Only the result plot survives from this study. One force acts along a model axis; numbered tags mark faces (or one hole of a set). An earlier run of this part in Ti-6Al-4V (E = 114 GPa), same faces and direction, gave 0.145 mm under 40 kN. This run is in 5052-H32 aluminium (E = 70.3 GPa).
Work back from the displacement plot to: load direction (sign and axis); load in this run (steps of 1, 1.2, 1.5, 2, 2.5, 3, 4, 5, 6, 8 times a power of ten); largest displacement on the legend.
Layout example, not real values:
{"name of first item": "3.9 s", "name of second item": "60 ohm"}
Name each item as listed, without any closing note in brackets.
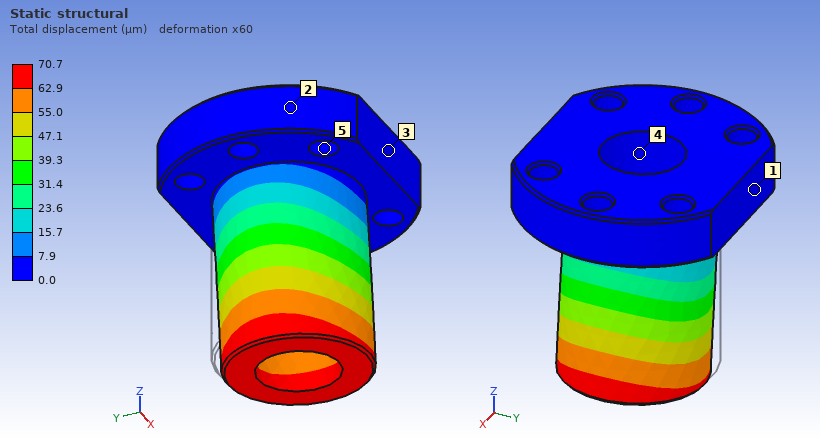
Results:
{"load direction": "+X", "load in this run": "12 kN", "largest displacement on the legend": "70.7 µm"}
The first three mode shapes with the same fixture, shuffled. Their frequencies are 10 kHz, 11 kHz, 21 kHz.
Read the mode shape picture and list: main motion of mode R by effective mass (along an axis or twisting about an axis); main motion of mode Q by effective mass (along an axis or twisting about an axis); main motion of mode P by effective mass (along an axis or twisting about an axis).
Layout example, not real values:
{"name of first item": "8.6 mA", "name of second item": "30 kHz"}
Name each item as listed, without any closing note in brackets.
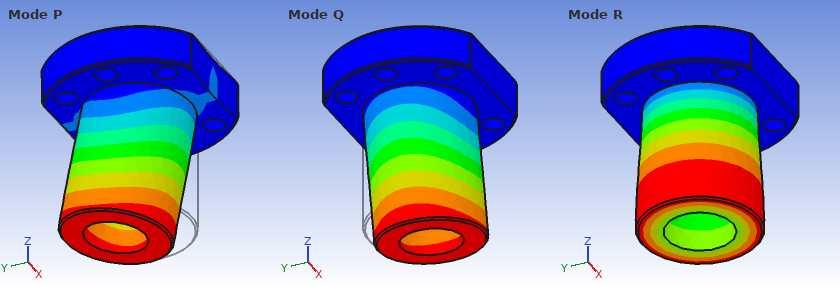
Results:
{"main motion of mode R by effective mass": "twisting about Z", "main motion of mode Q by effective mass": "along X", "main motion of mode P by effective mass": "along Y"}
